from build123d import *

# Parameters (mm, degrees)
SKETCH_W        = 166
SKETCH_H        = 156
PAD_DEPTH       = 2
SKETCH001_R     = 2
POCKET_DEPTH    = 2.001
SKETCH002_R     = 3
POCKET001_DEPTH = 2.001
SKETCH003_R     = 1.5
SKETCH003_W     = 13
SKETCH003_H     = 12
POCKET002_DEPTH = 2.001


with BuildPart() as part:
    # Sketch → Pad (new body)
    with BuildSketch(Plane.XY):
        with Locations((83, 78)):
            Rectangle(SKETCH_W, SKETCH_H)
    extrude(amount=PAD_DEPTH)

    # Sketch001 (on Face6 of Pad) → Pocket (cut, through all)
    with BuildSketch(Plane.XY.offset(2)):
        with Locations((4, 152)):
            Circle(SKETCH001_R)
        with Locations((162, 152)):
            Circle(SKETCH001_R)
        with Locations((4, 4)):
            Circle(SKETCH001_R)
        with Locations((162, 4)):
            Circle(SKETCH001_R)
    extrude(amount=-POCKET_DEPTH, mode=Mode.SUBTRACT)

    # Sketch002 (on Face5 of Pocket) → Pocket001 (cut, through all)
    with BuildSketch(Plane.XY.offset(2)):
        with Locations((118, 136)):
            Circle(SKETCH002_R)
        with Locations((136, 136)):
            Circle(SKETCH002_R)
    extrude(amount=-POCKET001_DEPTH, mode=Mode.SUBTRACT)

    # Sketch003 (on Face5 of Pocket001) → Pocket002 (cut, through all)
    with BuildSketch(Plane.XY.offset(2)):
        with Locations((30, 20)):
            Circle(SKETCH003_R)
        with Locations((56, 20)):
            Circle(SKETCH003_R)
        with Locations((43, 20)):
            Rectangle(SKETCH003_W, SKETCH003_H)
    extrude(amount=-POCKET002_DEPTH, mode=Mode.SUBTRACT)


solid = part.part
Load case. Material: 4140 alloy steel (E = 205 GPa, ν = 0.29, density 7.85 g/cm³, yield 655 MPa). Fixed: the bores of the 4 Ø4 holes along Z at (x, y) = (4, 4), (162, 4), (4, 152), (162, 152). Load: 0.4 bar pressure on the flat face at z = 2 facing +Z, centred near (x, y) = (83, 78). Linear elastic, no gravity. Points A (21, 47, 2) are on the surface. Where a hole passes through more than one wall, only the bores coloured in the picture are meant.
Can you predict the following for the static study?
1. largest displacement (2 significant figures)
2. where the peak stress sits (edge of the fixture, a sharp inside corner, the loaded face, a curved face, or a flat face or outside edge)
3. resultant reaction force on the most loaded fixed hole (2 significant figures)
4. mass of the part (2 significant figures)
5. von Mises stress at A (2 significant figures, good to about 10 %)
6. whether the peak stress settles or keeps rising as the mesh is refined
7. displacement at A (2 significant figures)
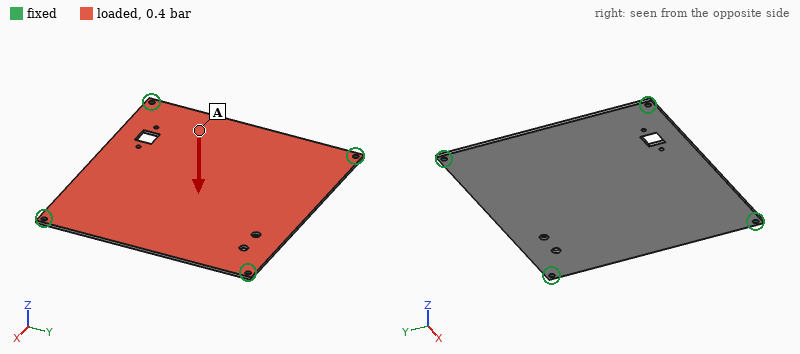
1.5 mm
edge of the fixture
260 N
400 g
62 MPa
keeps rising
0.74 mm
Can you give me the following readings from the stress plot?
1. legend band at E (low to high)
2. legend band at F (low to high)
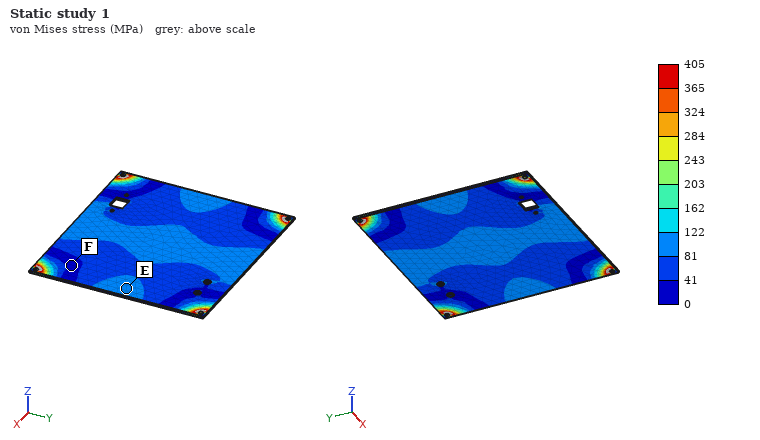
81 to 122 MPa
0 to 41 MPa
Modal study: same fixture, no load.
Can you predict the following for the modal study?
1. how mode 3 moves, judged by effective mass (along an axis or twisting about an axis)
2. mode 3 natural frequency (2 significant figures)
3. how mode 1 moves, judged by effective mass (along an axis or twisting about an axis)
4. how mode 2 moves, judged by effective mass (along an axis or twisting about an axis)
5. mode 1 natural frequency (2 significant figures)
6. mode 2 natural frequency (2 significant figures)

twisting about Y
490 Hz
along Z
twisting about X
250 Hz
460 Hz
